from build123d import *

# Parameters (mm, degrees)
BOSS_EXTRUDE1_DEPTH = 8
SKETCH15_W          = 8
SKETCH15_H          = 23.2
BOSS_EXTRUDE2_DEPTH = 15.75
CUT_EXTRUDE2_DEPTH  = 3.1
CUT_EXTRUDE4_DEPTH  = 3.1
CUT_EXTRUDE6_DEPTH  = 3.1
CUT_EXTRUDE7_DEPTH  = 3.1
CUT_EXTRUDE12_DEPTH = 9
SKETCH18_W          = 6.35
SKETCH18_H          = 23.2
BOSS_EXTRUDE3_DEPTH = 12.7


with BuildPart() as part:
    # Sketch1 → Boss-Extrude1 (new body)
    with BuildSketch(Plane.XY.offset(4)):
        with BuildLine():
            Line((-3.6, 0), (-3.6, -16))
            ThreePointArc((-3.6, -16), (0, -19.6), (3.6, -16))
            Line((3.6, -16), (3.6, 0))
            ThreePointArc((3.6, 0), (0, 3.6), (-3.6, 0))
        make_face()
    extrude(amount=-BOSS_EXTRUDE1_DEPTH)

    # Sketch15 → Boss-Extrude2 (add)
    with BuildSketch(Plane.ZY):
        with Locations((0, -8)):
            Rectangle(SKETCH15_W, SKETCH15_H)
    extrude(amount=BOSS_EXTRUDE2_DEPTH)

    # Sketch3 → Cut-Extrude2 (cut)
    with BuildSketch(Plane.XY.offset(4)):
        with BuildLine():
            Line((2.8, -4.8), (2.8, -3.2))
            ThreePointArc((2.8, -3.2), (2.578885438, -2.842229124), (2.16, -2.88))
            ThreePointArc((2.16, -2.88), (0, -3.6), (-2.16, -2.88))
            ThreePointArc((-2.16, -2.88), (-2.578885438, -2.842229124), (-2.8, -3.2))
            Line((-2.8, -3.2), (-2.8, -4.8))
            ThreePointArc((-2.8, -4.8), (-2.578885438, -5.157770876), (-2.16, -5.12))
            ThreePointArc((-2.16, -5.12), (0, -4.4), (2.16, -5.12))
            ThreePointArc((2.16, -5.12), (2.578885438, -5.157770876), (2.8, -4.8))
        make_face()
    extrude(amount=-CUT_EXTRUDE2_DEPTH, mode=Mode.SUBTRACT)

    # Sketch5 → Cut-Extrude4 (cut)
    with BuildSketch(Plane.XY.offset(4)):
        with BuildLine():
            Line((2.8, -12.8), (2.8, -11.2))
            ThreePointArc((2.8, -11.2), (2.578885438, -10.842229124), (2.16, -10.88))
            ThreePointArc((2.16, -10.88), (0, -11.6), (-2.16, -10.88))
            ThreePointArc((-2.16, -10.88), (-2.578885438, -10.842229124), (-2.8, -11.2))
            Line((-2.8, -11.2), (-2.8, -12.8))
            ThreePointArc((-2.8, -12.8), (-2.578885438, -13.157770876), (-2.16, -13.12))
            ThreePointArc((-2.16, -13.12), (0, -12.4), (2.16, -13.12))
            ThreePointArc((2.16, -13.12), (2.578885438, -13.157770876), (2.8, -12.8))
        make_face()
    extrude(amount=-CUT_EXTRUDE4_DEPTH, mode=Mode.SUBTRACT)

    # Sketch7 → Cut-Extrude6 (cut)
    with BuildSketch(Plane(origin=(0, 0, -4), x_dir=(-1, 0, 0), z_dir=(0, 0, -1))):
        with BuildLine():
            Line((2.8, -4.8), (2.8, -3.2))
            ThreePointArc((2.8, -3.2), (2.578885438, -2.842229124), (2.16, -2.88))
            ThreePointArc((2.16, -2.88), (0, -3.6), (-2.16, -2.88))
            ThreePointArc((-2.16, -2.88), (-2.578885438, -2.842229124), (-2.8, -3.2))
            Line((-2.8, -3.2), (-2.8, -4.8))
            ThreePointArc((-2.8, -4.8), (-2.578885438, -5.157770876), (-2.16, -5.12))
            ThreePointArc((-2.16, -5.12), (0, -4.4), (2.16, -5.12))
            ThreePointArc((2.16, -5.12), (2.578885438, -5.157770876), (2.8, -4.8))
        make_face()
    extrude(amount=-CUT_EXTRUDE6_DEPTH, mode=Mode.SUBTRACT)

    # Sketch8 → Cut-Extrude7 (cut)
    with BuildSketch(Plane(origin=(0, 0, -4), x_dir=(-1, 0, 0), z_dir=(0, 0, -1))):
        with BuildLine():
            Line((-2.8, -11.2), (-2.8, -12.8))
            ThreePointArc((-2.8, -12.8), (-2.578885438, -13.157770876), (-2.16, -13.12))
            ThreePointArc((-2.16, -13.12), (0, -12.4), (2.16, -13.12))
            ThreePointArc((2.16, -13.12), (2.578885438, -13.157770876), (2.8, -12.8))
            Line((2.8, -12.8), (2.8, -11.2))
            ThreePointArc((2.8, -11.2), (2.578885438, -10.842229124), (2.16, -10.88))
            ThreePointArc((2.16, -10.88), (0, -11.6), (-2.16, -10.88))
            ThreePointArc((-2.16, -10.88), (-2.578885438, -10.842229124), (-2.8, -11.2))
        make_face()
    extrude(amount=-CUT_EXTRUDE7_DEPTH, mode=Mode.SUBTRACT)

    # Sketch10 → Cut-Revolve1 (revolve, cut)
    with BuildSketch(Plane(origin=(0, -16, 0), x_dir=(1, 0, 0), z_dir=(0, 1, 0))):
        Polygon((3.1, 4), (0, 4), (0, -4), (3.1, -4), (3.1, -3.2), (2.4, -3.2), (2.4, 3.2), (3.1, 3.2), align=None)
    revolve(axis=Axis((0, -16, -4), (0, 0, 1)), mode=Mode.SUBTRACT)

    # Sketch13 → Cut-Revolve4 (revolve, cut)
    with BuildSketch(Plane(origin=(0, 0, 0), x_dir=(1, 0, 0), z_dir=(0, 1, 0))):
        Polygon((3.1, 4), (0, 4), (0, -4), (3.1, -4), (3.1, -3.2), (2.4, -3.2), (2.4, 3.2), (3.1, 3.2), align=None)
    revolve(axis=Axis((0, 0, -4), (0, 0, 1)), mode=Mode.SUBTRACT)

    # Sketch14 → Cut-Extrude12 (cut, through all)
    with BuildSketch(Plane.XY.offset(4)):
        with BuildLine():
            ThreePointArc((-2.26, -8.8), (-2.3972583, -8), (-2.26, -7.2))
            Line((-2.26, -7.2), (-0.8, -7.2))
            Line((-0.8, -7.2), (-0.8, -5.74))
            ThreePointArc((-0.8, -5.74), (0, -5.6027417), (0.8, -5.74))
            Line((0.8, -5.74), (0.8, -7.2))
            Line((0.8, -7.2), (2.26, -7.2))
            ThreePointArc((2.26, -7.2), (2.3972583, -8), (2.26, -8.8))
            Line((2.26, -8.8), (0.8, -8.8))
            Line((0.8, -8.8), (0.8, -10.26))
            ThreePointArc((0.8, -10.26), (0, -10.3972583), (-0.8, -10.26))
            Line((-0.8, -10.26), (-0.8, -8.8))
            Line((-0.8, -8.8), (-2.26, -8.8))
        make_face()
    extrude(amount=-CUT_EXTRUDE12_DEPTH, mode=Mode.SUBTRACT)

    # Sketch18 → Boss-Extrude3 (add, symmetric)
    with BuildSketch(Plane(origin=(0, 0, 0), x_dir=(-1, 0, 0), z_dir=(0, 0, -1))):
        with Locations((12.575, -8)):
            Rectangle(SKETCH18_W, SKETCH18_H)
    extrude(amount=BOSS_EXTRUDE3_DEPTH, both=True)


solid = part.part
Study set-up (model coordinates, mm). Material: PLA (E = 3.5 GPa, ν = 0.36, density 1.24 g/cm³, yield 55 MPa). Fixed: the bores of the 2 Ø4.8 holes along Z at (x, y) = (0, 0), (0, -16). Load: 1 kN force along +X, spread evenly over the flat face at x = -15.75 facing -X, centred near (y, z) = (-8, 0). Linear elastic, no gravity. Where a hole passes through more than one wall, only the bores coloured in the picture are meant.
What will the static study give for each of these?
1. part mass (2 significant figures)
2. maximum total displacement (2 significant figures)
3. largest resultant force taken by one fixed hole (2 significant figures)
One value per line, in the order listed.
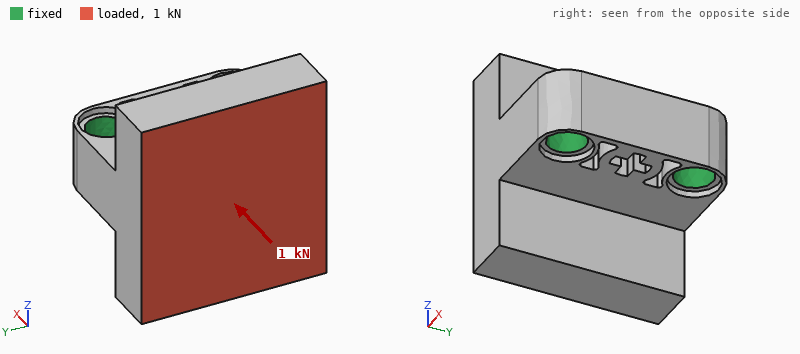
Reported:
6.9 g
73 µm
510 N
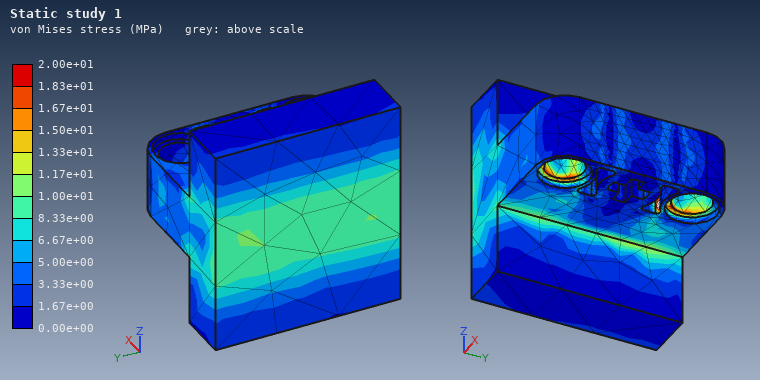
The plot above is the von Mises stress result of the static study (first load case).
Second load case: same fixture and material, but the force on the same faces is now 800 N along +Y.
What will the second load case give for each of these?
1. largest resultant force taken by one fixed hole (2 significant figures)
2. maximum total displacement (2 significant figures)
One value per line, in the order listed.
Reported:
740 N
0.10 mm
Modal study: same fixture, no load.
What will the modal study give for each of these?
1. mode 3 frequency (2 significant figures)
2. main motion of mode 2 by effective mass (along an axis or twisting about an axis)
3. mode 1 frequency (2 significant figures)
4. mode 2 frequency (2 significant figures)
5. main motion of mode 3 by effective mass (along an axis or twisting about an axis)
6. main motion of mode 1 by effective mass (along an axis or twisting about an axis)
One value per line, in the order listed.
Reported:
7900 Hz
twisting about X
3200 Hz
5800 Hz
along Y
along Z
